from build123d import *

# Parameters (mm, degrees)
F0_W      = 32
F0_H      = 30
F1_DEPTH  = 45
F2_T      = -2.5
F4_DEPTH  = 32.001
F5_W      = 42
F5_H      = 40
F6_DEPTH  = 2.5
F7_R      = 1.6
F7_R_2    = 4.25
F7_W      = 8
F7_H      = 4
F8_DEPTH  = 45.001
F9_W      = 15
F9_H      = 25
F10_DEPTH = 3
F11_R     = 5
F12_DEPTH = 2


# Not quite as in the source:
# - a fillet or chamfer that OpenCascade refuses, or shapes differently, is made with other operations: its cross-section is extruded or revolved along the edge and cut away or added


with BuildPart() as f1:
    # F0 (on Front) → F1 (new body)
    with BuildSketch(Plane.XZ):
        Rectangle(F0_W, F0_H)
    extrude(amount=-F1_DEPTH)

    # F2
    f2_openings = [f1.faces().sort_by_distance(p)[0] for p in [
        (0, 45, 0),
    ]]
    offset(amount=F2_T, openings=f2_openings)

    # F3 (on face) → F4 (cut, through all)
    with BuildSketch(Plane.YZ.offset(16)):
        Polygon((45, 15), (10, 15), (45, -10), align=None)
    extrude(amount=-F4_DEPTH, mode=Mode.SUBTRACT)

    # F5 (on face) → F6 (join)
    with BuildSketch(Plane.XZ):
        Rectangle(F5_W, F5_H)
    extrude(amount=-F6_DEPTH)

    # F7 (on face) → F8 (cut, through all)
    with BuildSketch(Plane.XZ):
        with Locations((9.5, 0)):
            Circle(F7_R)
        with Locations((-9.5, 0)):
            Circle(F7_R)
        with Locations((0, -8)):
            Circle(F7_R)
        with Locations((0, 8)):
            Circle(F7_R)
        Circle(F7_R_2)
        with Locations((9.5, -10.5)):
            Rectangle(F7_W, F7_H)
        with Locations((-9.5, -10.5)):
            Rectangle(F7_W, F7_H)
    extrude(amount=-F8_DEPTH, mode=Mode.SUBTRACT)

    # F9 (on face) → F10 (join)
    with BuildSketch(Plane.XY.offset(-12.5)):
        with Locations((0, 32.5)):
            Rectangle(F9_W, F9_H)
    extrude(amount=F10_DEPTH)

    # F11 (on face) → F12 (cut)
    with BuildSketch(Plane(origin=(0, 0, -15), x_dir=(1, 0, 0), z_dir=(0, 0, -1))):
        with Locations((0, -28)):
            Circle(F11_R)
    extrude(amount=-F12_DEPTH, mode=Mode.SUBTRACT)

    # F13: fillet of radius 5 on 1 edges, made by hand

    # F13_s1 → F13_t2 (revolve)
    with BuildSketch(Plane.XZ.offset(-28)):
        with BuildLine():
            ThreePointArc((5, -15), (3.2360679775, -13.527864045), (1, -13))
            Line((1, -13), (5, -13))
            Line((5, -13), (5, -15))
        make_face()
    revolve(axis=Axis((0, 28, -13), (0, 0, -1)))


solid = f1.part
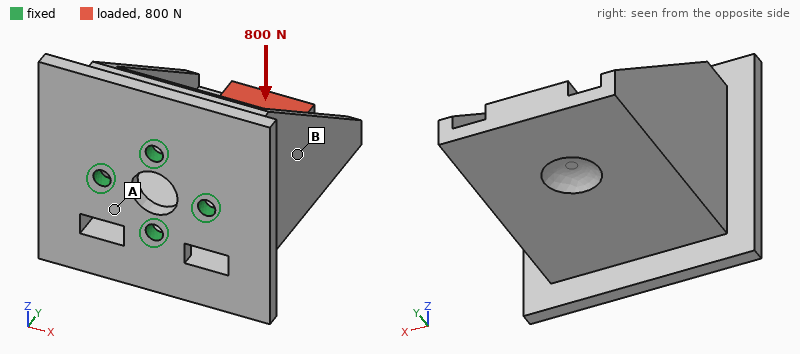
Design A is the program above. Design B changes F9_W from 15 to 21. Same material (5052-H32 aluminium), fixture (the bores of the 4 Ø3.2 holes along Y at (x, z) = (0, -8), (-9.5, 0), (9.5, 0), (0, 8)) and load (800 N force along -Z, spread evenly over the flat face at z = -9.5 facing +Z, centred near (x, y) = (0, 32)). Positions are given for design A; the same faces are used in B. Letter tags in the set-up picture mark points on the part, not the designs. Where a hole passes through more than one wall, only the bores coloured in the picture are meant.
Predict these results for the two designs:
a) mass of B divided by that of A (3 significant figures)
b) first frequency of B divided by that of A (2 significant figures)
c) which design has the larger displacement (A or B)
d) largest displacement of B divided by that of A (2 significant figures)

1.04
0.99
A
0.90
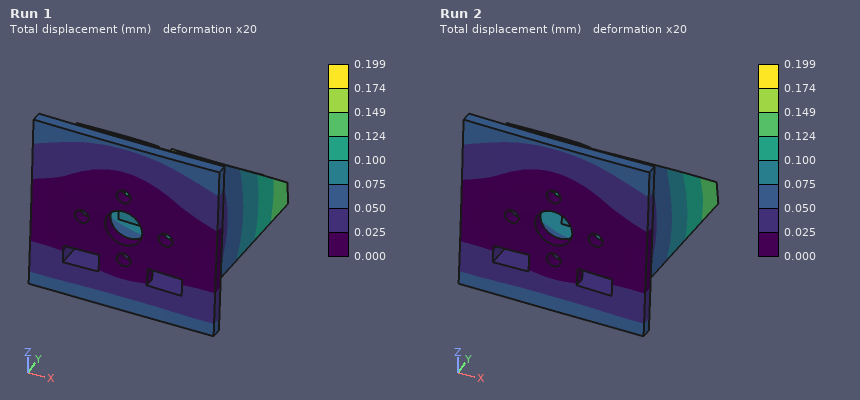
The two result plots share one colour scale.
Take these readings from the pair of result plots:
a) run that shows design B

Run 1
